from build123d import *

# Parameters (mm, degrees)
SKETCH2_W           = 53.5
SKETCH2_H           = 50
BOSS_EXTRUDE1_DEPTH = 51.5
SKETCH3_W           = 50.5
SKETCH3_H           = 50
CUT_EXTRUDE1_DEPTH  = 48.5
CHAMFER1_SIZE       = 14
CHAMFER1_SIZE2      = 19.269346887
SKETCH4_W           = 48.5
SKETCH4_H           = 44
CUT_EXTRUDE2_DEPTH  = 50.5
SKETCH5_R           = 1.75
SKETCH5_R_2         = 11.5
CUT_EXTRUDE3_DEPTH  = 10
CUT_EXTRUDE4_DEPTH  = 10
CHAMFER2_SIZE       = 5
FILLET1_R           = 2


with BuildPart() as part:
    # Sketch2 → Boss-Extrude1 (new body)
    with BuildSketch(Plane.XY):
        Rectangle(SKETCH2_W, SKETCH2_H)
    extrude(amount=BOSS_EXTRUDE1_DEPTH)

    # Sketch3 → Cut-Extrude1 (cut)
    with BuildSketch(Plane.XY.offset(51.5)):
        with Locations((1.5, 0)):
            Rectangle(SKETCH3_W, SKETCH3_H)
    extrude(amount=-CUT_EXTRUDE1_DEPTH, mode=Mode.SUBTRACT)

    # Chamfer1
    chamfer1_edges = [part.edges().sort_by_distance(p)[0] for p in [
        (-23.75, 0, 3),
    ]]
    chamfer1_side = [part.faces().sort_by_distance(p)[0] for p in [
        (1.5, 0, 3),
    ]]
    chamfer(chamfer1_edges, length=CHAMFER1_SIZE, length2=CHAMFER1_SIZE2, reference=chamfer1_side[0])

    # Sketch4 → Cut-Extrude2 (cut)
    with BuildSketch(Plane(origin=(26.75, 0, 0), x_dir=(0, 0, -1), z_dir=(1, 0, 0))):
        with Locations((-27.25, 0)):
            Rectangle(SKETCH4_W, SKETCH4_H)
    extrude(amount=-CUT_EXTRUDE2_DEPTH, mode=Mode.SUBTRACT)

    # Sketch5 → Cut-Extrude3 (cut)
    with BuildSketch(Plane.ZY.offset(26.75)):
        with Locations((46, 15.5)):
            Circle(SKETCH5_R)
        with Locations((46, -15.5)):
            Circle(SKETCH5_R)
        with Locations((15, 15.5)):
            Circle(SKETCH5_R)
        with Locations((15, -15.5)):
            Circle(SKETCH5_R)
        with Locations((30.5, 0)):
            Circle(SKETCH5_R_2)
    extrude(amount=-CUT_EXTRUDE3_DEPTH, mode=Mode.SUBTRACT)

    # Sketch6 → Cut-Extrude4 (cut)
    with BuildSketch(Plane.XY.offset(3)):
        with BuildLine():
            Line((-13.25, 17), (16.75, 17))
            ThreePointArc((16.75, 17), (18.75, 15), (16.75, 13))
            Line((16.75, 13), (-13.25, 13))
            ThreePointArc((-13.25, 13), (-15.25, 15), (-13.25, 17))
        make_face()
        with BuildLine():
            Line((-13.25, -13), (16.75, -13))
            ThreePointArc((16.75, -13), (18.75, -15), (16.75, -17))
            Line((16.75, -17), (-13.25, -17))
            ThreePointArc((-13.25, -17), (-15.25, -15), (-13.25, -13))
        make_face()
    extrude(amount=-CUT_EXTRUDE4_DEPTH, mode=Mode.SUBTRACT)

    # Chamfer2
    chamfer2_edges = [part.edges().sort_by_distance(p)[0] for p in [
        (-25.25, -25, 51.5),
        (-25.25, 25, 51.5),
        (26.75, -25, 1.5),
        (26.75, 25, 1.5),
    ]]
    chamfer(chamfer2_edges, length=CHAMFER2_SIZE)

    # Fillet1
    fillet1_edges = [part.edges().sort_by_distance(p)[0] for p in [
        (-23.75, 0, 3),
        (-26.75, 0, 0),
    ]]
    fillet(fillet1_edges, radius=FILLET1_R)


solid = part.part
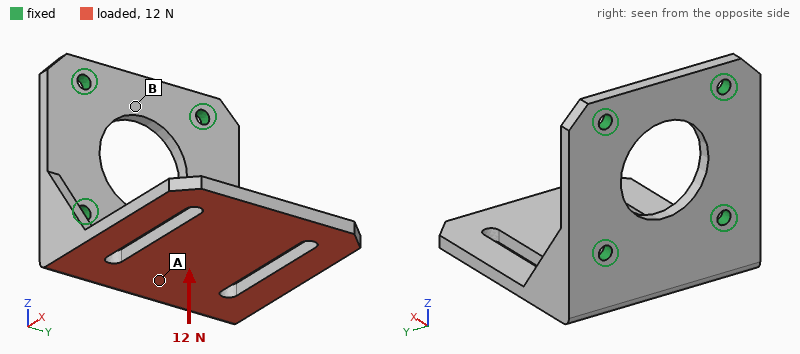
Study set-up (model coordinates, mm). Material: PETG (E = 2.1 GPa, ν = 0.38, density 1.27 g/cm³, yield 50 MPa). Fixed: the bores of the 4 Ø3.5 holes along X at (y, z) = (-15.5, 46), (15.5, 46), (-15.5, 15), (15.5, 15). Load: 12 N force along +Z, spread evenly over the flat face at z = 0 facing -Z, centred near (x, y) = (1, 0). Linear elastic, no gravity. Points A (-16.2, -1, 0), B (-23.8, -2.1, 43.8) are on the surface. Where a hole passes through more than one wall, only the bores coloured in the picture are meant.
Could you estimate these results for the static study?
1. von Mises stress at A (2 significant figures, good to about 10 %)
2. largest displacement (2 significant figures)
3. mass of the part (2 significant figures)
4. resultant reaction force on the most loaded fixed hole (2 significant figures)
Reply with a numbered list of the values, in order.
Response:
1. 1.6 MPa
2. 0.91 mm
3. 18 g
4. 6.2 N
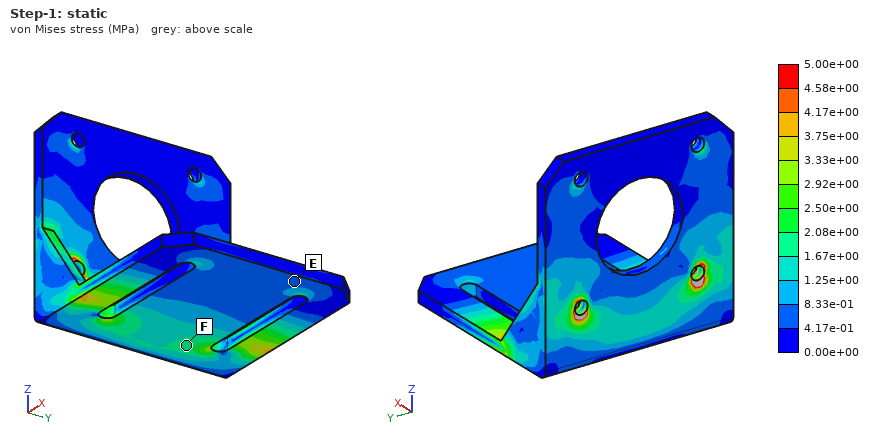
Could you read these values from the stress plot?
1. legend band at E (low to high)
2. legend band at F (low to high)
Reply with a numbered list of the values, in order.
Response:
1. 4.17e-01 to 8.33e-01 MPa
2. 1.67e+00 to 2.08e+00 MPa
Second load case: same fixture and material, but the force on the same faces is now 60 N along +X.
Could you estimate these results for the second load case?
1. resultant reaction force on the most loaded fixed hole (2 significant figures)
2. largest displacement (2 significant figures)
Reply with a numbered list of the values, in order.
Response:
1. 35 N
2. 1.0 mm
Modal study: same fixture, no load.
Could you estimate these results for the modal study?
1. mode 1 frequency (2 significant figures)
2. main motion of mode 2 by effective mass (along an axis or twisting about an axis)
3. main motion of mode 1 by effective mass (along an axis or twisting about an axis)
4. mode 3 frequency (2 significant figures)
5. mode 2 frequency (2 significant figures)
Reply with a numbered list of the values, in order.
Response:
1. 240 Hz
2. along Y
3. along Z
4. 830 Hz
5. 530 Hz
